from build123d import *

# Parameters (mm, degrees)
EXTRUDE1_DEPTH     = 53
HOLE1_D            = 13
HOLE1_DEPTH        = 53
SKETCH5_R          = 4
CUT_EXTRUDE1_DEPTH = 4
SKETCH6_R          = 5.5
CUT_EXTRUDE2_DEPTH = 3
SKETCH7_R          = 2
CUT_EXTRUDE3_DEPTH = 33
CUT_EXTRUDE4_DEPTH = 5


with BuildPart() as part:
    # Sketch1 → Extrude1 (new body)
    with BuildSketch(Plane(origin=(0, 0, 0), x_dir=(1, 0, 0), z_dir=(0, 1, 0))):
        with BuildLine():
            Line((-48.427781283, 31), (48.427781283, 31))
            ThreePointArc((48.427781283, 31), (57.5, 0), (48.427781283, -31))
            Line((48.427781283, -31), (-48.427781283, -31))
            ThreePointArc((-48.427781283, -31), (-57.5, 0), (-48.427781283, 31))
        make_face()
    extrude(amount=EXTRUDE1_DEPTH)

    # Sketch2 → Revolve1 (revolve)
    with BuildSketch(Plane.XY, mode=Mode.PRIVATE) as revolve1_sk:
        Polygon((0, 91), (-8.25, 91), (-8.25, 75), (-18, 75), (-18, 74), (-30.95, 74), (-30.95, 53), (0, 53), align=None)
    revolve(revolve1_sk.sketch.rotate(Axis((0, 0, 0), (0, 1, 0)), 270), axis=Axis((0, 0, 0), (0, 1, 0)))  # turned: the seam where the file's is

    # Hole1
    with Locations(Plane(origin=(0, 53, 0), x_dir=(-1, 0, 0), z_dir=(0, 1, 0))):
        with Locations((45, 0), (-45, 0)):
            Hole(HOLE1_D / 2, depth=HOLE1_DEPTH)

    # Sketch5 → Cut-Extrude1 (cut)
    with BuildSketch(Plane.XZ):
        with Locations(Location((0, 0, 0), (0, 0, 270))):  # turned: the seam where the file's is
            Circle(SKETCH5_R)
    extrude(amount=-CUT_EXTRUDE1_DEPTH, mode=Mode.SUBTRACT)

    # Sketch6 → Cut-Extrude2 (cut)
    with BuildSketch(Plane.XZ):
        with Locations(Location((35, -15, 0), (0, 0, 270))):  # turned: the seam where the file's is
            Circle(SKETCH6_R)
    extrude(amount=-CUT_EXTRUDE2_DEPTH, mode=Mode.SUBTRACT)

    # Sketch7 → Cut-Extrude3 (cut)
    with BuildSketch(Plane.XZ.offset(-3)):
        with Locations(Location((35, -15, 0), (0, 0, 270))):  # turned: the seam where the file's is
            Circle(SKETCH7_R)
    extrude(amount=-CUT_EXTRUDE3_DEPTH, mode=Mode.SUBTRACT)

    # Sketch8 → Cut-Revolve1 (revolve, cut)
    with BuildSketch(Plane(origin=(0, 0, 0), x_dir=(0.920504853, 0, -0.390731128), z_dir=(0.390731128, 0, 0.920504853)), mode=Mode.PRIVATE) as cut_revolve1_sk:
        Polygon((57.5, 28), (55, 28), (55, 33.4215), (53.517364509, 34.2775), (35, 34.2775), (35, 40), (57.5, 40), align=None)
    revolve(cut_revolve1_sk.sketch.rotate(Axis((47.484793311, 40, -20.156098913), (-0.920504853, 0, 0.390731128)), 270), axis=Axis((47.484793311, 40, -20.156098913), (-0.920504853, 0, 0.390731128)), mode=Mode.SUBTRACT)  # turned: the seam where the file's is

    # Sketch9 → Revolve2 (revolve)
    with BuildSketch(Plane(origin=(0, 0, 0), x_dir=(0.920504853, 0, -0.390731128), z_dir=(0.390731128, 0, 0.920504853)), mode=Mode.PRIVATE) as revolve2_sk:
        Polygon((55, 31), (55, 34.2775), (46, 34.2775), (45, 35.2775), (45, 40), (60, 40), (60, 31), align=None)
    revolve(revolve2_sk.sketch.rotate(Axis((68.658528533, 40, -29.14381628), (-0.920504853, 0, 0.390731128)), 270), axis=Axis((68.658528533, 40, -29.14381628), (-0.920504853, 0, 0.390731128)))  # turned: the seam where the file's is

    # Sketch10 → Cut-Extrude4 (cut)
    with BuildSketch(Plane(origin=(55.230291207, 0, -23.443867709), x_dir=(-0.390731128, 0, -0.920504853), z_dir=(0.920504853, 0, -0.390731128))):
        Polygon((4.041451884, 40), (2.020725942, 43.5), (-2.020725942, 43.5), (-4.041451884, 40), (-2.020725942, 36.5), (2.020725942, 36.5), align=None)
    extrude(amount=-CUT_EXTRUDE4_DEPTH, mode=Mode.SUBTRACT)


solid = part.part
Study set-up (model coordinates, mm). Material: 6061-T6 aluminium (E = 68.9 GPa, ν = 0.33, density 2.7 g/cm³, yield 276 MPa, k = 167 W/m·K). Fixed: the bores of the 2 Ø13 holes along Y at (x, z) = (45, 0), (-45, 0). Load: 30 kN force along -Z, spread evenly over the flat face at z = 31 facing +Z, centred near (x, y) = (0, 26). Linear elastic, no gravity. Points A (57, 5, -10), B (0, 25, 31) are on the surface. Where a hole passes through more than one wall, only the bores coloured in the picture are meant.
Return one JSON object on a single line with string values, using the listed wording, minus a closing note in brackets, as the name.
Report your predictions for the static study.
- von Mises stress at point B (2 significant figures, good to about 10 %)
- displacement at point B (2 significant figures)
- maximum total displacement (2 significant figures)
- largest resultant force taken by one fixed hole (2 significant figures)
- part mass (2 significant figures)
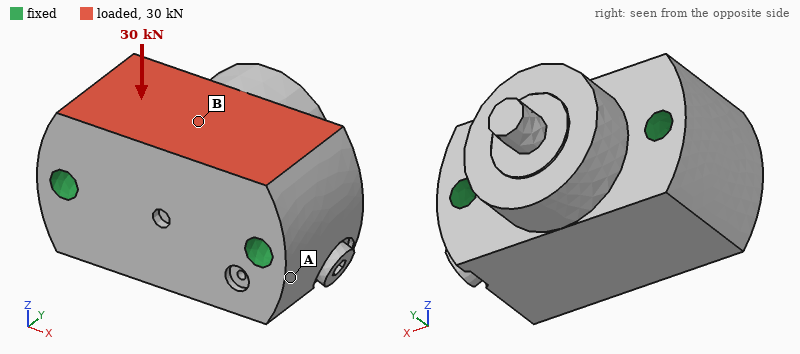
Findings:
{"von Mises stress at point B": "7.2 MPa", "displacement at point B": "7.1 µm", "maximum total displacement": "8.2 µm", "largest resultant force taken by one fixed hole": "15 kN", "part mass": "1.1 kg"}
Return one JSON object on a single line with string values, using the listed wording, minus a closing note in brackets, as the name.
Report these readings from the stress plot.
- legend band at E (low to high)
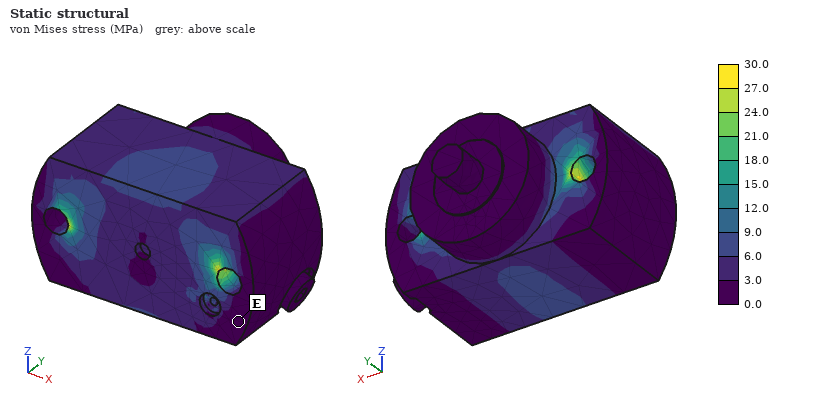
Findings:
{"legend band at E": "0.0 to 3.0 MPa"}
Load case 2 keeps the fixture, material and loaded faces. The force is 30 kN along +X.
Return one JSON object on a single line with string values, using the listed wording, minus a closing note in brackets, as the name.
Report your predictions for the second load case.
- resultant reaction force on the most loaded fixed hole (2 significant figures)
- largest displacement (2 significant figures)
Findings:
{"resultant reaction force on the most loaded fixed hole": "18 kN", "largest displacement": "8.7 µm"}
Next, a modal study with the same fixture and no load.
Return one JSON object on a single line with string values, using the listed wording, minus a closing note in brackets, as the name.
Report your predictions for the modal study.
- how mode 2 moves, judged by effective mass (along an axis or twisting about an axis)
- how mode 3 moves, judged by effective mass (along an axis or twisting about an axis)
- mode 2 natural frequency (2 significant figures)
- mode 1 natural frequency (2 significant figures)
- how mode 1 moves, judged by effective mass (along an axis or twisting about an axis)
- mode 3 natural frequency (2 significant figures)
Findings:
{"how mode 2 moves, judged by effective mass": "along Y", "how mode 3 moves, judged by effective mass": "along Z", "mode 2 natural frequency": "12 kHz", "mode 1 natural frequency": "8500 Hz", "how mode 1 moves, judged by effective mass": "along Z", "mode 3 natural frequency": "13 kHz"}
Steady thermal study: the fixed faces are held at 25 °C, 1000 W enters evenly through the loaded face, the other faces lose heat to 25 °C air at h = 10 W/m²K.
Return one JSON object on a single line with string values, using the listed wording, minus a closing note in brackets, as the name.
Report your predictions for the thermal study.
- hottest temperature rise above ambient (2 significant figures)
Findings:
{"hottest temperature rise above ambient": "48 K"}
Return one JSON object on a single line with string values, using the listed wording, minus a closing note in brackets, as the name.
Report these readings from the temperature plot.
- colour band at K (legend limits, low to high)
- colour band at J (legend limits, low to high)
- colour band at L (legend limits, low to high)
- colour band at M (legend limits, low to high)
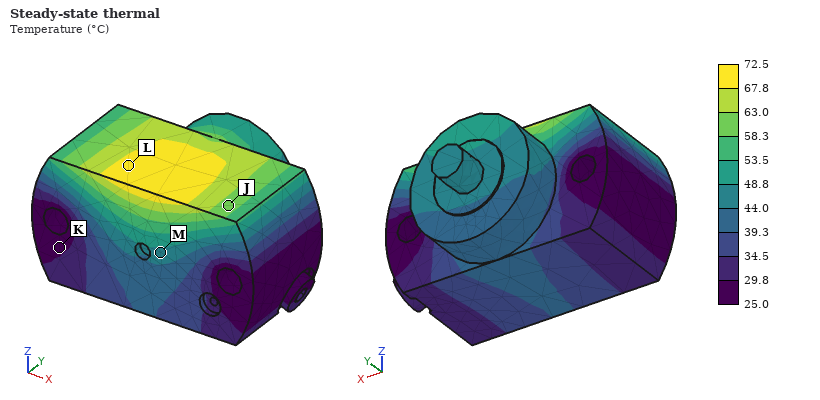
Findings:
{"colour band at K": "25.0 to 29.8 °C", "colour band at J": "58.3 to 63.0 °C", "colour band at L": "67.8 to 72.5 °C", "colour band at M": "44.0 to 48.8 °C"}
